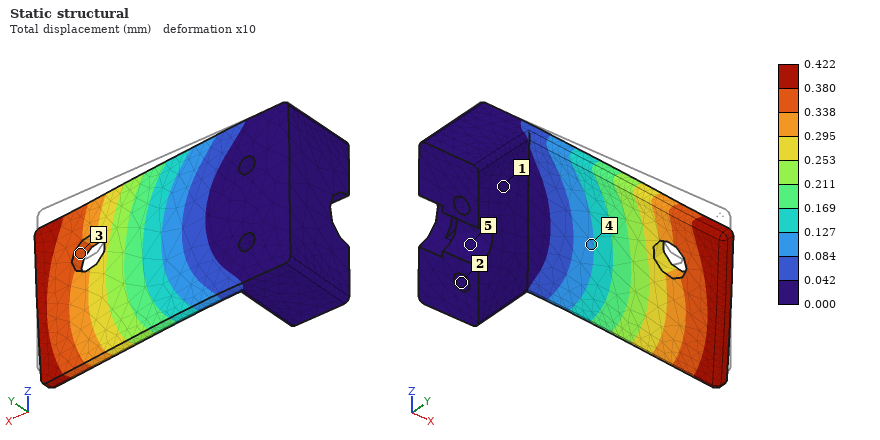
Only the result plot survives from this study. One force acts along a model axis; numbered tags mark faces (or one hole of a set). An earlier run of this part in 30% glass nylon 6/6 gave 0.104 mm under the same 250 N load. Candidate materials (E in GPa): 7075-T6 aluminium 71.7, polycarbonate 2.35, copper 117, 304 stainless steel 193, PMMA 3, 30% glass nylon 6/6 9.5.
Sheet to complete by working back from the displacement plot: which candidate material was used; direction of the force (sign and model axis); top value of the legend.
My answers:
polycarbonate
-Z
0.422 mm
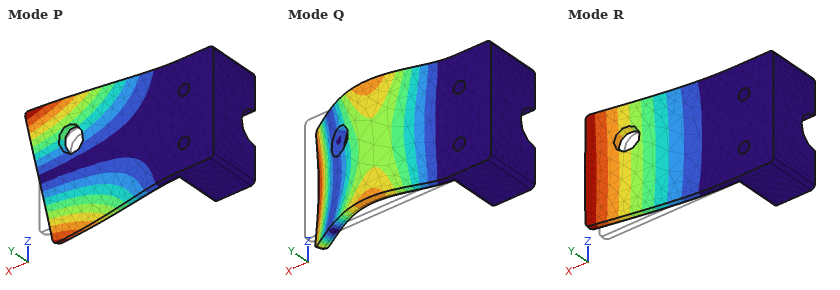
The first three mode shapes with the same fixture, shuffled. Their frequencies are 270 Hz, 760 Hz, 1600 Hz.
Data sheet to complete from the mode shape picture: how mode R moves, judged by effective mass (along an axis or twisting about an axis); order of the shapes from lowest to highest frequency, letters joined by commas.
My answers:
along Y
R, P, Q
